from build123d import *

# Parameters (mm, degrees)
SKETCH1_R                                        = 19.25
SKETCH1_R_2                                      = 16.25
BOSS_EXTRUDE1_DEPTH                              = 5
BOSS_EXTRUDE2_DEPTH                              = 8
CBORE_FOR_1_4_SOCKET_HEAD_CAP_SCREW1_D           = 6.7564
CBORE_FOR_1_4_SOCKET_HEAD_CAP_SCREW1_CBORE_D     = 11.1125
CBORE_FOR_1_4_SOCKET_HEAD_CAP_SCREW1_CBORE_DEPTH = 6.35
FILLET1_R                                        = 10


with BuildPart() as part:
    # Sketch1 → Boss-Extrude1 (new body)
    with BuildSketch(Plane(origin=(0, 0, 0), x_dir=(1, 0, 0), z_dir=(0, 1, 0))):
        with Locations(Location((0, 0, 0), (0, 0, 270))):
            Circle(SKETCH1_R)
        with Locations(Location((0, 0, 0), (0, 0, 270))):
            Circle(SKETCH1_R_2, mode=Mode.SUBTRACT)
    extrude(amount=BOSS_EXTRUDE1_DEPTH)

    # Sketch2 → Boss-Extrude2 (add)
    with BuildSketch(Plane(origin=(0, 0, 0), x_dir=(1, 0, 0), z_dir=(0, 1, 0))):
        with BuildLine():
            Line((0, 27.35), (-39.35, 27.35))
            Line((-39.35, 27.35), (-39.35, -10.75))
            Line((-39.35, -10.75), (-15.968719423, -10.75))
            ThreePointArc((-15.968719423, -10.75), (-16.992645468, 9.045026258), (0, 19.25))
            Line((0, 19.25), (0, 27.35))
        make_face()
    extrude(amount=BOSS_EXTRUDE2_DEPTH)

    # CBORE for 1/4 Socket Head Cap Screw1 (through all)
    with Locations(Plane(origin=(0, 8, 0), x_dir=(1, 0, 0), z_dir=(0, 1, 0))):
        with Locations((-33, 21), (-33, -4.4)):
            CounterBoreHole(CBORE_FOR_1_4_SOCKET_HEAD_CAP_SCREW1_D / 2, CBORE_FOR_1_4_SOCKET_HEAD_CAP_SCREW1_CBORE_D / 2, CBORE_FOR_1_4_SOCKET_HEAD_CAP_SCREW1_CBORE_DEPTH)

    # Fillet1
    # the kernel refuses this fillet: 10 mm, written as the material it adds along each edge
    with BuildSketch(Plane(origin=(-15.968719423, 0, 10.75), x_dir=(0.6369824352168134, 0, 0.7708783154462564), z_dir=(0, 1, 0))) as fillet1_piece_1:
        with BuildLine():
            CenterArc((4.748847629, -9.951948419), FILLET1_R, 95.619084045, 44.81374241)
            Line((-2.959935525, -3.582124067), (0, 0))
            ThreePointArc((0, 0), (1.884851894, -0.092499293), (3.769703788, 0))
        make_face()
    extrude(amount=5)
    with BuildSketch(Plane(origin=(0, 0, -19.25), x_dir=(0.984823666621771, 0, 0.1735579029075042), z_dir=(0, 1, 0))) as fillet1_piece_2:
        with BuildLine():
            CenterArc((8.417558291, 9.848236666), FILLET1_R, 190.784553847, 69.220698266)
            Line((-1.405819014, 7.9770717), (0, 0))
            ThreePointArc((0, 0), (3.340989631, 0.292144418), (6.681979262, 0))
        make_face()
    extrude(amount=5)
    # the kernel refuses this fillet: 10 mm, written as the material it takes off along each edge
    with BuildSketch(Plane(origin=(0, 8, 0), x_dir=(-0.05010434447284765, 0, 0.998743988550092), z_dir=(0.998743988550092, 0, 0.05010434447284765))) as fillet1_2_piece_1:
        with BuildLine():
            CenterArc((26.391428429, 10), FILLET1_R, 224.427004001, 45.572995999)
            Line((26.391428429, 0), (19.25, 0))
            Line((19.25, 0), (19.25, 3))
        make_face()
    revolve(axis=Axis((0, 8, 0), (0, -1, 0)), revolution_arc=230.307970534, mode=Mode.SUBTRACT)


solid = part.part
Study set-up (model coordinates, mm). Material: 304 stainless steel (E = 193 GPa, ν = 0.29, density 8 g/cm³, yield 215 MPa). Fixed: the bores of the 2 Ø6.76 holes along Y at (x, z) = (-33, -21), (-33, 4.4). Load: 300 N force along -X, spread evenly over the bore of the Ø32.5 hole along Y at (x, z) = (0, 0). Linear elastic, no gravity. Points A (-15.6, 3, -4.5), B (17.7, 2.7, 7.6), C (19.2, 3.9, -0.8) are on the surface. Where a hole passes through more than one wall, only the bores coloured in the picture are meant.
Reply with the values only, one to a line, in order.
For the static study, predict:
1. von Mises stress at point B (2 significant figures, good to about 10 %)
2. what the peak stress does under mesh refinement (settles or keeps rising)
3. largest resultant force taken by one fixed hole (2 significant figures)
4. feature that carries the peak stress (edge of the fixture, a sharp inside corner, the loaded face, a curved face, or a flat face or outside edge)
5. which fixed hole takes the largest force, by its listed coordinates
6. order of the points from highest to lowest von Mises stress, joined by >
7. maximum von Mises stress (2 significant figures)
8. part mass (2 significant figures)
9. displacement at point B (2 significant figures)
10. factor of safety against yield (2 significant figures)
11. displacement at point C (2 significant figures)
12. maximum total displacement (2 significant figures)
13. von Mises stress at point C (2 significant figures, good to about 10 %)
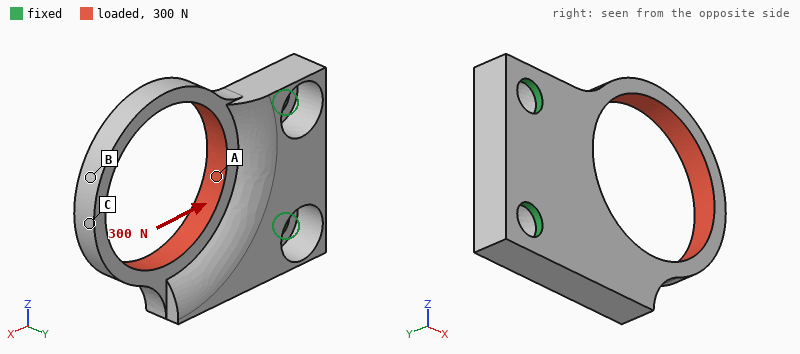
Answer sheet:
17 MPa
settles
240 N
a curved face
(-33, 4.4)
C > B > A
58 MPa
66 g
17 µm
3.7
18 µm
19 µm
24 MPa
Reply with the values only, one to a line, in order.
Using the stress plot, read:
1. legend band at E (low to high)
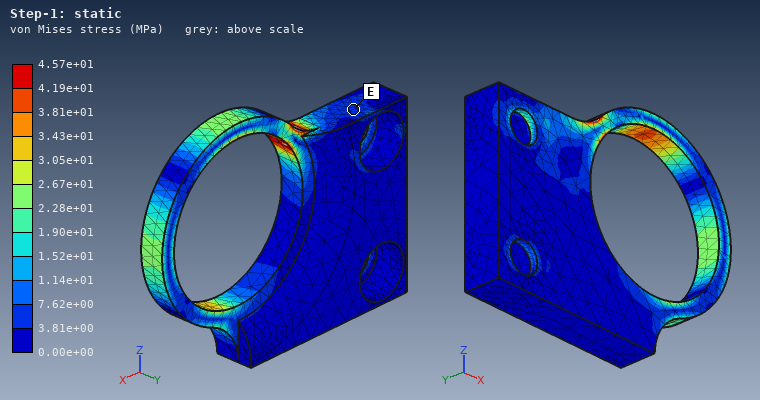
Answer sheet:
3.81e+00 to 7.62e+00 MPa
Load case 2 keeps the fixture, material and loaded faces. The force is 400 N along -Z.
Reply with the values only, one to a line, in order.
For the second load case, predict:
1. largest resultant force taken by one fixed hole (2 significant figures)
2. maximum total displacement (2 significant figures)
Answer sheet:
500 N
42 µm
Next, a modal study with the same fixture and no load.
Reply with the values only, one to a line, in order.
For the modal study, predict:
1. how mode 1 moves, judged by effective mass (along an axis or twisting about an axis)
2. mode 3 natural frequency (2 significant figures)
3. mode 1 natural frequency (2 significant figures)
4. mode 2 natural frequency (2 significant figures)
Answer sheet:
along Y
4400 Hz
2100 Hz
4300 Hz
